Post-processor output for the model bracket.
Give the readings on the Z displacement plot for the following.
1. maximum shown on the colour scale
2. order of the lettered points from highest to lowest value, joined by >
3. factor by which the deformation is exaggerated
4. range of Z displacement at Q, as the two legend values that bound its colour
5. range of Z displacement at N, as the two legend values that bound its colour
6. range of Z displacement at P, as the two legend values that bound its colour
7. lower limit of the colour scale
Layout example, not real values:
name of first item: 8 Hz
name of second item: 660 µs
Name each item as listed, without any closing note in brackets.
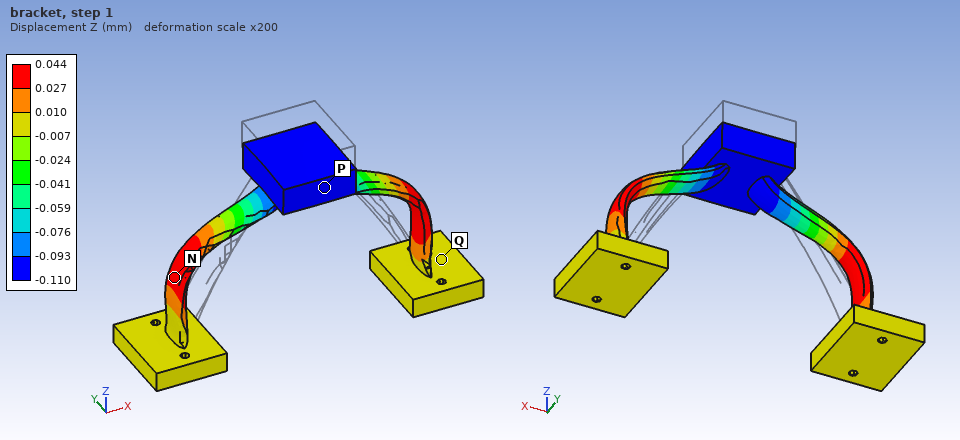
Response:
maximum shown on the colour scale: 0.044 mm
order of the lettered points from highest to lowest value, joined by >: N > Q > P
factor by which the deformation is exaggerated: 200
range of Z displacement at Q, as the two legend values that bound its colour: -0.007 to 0.010 mm
range of Z displacement at N, as the two legend values that bound its colour: 0.027 to 0.044 mm
range of Z displacement at P, as the two legend values that bound its colour: -0.110 to -0.093 mm
lower limit of the colour scale: -0.110 mm
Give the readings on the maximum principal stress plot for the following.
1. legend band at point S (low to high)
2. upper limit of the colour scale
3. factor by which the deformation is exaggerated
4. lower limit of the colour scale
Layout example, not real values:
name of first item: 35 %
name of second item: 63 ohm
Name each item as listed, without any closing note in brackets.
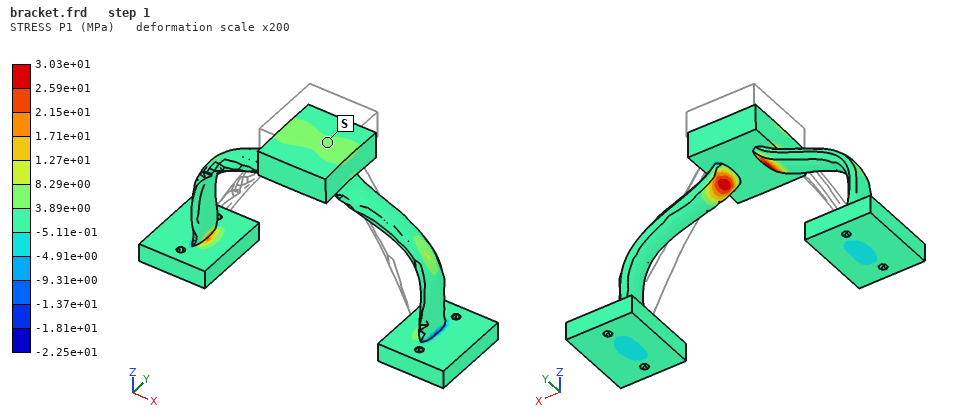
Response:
legend band at point S: 3.89e+00 to 8.29e+00 MPa
upper limit of the colour scale: 3.03e+01 MPa
factor by which the deformation is exaggerated: 200
lower limit of the colour scale: -2.25e+01 MPa
